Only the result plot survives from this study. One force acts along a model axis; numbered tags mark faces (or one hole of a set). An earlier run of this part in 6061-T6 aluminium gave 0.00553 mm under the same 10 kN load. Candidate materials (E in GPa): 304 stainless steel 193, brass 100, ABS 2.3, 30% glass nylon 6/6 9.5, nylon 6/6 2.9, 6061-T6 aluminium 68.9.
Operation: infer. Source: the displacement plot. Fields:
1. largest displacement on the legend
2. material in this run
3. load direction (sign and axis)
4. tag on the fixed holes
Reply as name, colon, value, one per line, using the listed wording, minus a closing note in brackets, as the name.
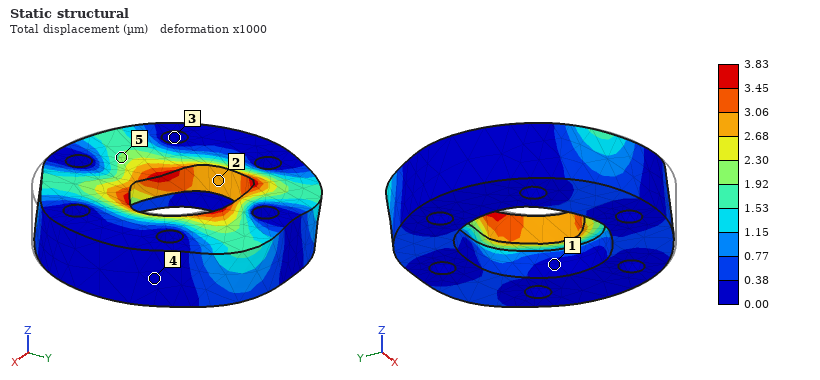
largest displacement on the legend: 3.83 µm
material in this run: brass
load direction: +Y
tag on the fixed holes: 3
